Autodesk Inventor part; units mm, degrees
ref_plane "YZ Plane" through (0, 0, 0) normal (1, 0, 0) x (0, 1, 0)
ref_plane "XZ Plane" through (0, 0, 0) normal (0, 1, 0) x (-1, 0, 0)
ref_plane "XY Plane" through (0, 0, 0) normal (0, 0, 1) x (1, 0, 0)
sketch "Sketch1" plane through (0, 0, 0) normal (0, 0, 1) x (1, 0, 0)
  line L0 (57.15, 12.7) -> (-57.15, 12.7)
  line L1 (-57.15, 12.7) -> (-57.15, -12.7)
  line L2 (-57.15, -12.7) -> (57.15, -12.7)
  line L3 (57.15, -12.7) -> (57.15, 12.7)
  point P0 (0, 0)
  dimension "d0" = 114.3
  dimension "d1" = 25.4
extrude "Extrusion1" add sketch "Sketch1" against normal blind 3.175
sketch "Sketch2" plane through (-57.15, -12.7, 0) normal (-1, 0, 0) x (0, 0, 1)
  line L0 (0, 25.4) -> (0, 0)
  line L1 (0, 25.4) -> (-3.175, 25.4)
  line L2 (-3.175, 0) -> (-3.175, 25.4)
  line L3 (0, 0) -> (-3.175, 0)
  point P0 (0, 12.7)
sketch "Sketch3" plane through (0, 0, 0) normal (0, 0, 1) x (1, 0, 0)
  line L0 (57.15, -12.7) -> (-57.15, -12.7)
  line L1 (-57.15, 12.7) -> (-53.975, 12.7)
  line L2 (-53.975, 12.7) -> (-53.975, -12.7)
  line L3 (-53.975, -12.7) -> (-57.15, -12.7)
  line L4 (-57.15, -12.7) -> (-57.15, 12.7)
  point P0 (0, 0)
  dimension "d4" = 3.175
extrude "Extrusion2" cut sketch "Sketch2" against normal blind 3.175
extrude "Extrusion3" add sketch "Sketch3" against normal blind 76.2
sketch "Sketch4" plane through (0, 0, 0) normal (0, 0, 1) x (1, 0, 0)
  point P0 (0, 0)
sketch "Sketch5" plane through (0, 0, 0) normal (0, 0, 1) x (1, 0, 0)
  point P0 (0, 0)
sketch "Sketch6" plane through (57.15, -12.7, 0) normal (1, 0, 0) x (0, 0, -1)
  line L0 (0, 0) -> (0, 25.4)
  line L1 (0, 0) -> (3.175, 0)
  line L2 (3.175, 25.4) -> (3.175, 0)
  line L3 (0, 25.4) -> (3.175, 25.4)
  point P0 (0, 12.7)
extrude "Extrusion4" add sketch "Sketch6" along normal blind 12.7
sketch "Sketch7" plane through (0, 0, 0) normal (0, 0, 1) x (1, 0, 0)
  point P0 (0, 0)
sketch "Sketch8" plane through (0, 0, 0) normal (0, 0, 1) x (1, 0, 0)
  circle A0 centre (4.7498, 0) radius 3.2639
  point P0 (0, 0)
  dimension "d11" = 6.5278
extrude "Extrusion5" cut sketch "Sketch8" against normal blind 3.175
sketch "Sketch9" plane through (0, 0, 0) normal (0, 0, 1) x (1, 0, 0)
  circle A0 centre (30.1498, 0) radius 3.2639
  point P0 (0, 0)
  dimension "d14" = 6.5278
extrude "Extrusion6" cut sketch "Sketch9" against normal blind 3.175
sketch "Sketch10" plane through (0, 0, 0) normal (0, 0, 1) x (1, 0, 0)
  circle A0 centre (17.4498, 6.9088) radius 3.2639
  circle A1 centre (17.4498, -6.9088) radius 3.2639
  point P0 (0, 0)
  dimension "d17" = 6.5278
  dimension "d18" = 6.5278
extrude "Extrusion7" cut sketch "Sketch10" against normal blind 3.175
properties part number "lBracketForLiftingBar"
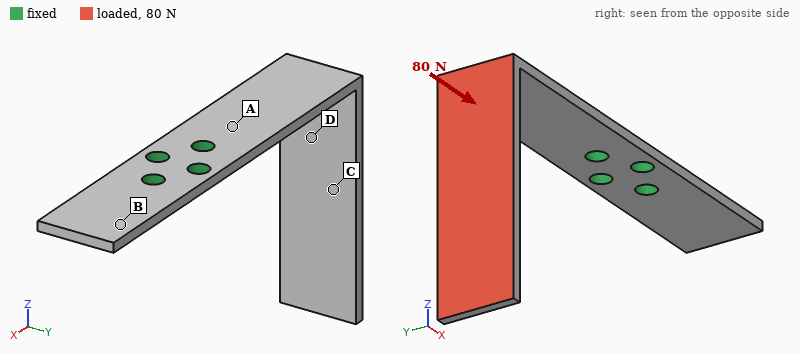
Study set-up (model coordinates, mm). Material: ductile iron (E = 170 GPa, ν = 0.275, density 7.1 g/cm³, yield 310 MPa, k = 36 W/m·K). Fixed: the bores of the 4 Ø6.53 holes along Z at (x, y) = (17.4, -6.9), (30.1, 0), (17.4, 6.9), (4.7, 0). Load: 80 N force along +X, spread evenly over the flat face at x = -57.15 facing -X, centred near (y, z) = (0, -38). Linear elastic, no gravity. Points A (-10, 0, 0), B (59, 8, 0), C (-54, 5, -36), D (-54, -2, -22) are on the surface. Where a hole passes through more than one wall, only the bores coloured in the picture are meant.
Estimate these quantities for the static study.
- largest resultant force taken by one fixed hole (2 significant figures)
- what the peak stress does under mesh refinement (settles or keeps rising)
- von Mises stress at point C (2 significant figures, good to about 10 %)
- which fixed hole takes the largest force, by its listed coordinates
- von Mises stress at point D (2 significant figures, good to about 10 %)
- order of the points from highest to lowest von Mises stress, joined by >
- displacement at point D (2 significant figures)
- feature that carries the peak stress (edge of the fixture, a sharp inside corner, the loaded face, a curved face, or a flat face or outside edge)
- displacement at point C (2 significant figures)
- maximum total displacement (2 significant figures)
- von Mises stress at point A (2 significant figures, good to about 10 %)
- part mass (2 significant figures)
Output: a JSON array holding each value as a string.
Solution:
["100 N", "keeps rising", "20 MPa", "(4.7, 0)", "35 MPa", "A > D > C > B", "0.52 mm", "edge of the fixture", "0.72 mm", "1.5 mm", "62 MPa", "110 g"]
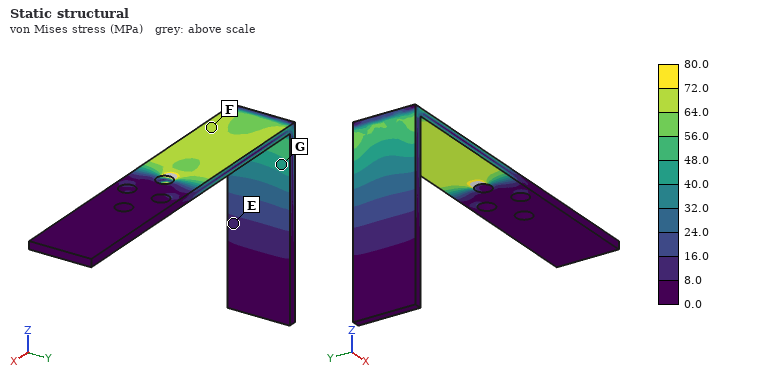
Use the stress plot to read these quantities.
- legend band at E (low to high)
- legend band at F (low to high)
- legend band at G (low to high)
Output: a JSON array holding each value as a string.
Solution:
["8.0 to 16.0 MPa", "64.0 to 72.0 MPa", "40.0 to 48.0 MPa"]
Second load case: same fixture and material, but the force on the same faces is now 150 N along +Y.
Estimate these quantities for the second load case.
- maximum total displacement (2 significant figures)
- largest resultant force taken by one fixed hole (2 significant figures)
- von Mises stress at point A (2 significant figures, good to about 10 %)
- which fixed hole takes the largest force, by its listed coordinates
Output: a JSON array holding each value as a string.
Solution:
["1.4 mm", "330 N", "110 MPa", "(4.7, 0)"]
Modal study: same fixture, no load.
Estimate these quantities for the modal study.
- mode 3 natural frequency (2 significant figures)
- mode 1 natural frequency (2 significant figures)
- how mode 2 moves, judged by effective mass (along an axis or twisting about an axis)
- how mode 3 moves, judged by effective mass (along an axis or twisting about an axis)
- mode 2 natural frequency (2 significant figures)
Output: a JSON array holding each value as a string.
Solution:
["530 Hz", "190 Hz", "along Y", "along Z", "300 Hz"]
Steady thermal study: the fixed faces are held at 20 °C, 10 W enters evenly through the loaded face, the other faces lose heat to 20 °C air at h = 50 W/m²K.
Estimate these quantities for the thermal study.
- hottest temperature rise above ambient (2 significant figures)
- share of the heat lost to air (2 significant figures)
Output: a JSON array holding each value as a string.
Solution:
["63 K", "90 %"]
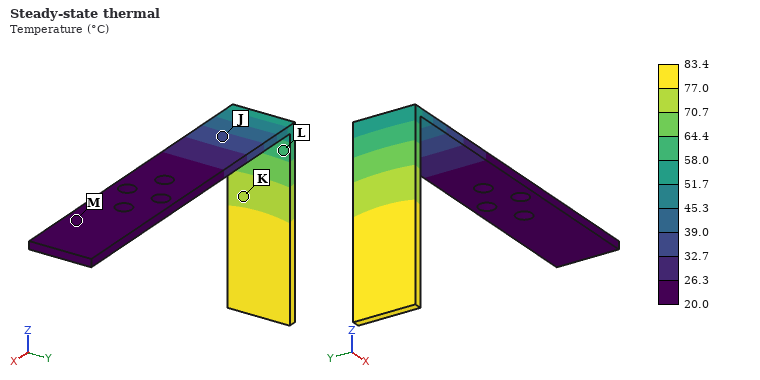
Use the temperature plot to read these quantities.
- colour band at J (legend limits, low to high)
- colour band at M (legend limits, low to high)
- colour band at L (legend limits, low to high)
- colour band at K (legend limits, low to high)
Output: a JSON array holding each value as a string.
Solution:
["32.7 to 39.0 °C", "20.0 to 26.3 °C", "58.0 to 64.4 °C", "70.7 to 77.0 °C"]
